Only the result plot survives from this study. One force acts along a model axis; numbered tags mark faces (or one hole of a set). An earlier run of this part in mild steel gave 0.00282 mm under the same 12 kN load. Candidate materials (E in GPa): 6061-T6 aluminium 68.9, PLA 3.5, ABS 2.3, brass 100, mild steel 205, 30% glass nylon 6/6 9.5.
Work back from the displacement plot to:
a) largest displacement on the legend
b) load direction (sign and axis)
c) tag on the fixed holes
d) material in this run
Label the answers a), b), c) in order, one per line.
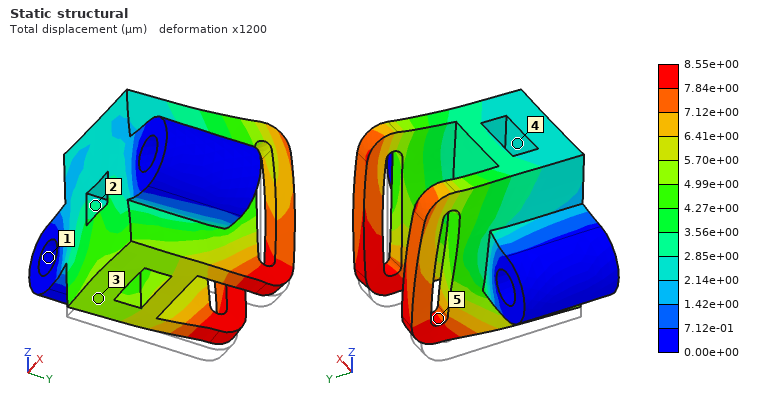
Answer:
a) 8.55e+00 µm
b) +Z
c) 1
d) 6061-T6 aluminium
